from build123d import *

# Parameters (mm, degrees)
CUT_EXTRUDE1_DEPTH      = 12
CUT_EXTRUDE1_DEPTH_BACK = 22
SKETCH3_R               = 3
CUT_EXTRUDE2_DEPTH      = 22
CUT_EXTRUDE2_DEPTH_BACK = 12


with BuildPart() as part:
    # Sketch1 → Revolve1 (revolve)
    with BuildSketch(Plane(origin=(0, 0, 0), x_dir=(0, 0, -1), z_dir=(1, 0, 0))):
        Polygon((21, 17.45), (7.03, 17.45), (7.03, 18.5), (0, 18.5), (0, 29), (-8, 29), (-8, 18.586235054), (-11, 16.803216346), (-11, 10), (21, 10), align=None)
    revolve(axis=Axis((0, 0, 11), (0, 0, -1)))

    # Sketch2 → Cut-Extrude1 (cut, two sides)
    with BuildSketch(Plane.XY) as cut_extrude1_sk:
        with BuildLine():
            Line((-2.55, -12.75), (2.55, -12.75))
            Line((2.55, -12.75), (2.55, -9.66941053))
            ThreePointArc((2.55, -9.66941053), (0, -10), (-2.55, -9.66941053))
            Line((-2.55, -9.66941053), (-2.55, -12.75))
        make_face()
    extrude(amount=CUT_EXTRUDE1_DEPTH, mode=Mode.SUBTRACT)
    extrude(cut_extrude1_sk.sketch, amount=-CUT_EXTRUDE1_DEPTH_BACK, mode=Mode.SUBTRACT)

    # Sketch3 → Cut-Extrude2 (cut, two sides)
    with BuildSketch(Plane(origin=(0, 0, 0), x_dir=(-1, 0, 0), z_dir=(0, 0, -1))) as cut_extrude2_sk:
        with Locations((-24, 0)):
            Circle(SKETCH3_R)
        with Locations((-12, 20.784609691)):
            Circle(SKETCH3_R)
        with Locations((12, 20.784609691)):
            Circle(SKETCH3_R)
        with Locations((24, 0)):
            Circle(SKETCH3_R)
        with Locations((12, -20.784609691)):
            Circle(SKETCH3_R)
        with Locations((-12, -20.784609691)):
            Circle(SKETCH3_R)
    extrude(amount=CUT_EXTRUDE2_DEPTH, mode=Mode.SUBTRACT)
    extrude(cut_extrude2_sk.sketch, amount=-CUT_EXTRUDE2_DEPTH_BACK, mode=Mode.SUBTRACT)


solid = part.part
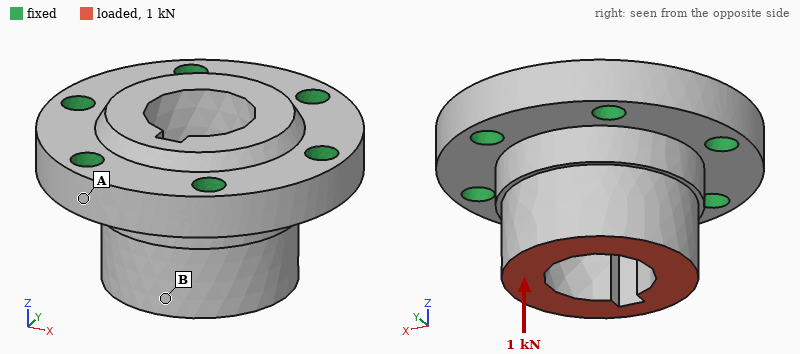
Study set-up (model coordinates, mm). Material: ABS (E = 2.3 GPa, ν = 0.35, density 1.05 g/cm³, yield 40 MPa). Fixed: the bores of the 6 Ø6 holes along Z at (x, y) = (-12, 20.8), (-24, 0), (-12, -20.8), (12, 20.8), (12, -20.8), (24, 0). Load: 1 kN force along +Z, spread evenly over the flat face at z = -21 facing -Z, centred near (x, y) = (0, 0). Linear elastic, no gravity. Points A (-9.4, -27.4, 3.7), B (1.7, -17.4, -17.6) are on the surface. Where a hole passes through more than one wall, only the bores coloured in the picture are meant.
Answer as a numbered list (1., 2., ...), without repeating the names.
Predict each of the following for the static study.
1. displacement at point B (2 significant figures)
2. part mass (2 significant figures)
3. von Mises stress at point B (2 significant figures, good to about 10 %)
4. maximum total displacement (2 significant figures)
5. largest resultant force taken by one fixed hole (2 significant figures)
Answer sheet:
1. 26 µm
2. 35 g
3. 1.6 MPa
4. 29 µm
5. 180 N
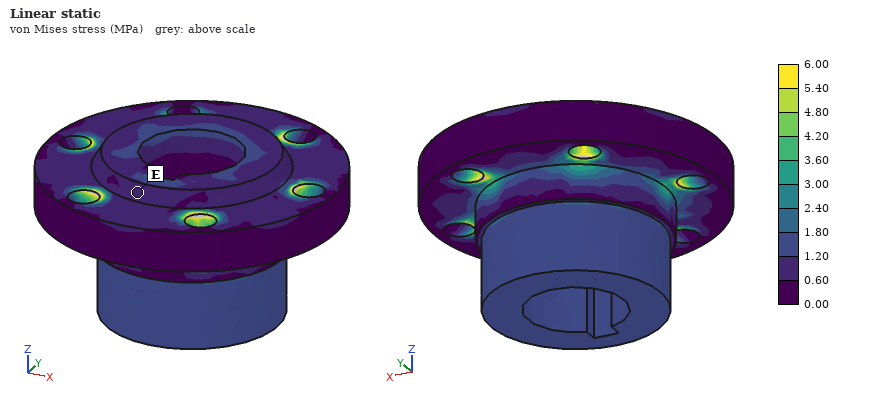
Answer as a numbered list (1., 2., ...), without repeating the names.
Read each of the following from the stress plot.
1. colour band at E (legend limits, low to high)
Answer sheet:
1. 0.60 to 1.20 MPa
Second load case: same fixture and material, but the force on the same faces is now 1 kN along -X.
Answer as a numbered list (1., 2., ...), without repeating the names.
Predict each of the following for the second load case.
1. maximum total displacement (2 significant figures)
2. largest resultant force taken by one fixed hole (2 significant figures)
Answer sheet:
1. 0.16 mm
2. 450 N
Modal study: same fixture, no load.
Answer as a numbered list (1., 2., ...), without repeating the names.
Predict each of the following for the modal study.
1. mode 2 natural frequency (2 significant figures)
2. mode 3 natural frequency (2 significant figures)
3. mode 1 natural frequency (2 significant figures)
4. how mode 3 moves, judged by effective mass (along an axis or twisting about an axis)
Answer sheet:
1. 6100 Hz
2. 7800 Hz
3. 6000 Hz
4. along Z
